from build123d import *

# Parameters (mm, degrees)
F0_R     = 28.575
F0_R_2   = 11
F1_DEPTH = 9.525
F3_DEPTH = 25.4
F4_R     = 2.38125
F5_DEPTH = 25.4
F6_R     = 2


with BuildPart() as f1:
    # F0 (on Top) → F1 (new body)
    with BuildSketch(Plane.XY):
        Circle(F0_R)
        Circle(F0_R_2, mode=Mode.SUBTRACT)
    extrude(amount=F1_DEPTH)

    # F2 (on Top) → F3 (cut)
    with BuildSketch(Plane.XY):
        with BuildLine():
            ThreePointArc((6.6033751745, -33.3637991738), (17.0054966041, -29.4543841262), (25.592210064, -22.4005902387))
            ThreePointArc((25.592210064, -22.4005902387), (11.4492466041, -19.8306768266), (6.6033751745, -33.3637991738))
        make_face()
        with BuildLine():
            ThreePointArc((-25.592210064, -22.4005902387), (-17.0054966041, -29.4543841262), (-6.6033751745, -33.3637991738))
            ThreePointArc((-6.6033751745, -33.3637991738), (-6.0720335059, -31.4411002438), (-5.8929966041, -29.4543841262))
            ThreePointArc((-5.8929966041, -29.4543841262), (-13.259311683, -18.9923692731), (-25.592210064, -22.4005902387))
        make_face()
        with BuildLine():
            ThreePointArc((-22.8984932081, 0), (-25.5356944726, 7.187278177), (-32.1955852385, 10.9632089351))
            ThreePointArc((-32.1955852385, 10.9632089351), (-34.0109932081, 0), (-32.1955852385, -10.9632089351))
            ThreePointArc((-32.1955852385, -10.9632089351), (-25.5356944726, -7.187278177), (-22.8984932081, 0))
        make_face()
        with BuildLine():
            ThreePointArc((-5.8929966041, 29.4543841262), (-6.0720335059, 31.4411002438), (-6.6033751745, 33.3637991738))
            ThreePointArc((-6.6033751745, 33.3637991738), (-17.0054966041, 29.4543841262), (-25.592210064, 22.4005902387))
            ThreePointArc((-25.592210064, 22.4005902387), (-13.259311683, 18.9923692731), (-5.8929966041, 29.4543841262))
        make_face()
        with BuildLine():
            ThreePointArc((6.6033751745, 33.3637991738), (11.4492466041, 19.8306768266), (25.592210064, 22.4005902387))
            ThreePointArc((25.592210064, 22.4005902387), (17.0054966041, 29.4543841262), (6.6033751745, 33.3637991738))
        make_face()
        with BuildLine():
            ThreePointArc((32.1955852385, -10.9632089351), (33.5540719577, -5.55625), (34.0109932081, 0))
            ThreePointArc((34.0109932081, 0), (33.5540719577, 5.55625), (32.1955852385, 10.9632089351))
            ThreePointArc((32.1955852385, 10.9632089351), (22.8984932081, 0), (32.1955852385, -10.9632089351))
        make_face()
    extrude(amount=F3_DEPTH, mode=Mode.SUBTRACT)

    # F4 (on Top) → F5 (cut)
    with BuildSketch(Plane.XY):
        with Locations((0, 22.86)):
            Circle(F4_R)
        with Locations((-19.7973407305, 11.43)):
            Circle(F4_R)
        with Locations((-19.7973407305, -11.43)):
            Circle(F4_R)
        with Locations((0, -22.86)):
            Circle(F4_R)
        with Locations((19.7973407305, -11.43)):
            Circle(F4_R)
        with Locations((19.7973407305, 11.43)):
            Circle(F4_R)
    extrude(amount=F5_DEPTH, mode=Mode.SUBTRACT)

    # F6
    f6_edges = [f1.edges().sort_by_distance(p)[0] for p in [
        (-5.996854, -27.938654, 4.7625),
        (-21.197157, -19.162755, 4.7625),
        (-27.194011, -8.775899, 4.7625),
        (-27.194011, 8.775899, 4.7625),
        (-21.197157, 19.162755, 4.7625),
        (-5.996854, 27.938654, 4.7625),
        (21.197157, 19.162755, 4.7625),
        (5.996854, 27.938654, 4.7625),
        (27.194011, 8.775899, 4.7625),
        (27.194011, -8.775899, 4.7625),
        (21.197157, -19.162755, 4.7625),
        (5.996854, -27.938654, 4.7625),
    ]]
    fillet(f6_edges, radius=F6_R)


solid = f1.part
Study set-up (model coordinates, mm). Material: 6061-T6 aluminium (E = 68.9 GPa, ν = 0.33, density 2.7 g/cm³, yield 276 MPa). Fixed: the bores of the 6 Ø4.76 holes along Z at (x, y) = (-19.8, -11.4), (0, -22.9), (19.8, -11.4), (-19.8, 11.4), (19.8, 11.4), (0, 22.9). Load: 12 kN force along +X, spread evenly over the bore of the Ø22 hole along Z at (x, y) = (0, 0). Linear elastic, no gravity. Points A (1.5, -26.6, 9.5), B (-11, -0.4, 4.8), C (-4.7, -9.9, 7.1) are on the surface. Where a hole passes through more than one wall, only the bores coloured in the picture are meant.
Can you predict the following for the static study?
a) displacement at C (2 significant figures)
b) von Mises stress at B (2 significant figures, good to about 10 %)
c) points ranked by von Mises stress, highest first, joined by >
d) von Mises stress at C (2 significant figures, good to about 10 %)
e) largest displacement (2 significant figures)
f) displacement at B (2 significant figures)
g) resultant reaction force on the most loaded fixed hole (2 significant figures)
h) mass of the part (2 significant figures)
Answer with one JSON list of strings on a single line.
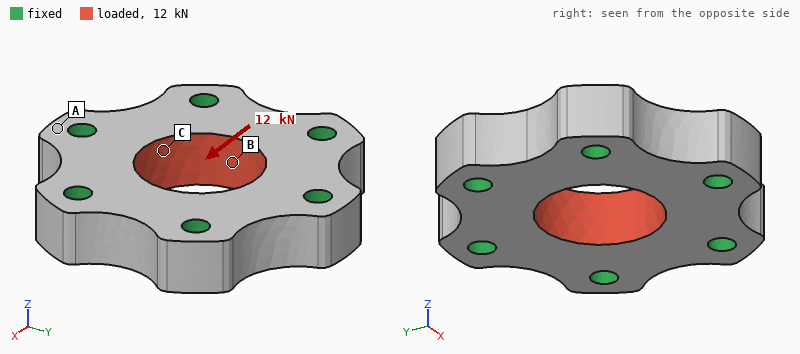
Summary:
["4.3 µm", "15 MPa", "C > B > A", "30 MPa", "4.8 µm", "4.6 µm", "2.7 kN", "43 g"]
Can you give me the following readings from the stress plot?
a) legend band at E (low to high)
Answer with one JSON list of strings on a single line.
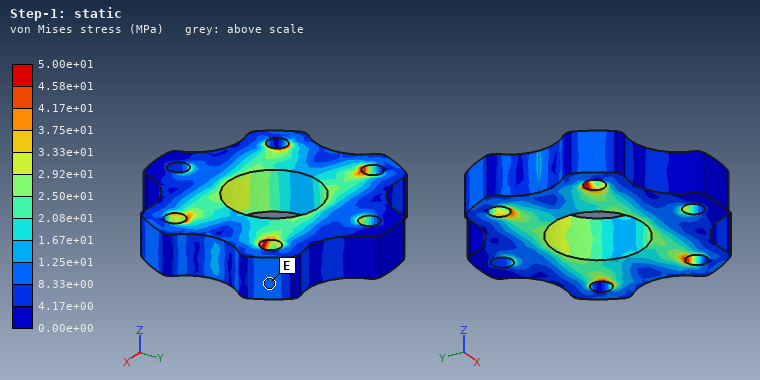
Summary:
["8.33e+00 to 1.25e+01 MPa"]
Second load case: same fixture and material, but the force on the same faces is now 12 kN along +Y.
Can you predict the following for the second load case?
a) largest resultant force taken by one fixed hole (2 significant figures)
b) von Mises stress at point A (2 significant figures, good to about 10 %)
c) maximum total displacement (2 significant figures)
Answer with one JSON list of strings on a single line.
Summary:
["3.1 kN", "8.6 MPa", "4.7 µm"]
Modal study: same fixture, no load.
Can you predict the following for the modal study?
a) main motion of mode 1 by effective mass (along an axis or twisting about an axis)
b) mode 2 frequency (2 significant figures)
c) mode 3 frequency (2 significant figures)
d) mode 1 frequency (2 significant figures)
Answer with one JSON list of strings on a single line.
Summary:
["along Z", "49 kHz", "49 kHz", "42 kHz"]
